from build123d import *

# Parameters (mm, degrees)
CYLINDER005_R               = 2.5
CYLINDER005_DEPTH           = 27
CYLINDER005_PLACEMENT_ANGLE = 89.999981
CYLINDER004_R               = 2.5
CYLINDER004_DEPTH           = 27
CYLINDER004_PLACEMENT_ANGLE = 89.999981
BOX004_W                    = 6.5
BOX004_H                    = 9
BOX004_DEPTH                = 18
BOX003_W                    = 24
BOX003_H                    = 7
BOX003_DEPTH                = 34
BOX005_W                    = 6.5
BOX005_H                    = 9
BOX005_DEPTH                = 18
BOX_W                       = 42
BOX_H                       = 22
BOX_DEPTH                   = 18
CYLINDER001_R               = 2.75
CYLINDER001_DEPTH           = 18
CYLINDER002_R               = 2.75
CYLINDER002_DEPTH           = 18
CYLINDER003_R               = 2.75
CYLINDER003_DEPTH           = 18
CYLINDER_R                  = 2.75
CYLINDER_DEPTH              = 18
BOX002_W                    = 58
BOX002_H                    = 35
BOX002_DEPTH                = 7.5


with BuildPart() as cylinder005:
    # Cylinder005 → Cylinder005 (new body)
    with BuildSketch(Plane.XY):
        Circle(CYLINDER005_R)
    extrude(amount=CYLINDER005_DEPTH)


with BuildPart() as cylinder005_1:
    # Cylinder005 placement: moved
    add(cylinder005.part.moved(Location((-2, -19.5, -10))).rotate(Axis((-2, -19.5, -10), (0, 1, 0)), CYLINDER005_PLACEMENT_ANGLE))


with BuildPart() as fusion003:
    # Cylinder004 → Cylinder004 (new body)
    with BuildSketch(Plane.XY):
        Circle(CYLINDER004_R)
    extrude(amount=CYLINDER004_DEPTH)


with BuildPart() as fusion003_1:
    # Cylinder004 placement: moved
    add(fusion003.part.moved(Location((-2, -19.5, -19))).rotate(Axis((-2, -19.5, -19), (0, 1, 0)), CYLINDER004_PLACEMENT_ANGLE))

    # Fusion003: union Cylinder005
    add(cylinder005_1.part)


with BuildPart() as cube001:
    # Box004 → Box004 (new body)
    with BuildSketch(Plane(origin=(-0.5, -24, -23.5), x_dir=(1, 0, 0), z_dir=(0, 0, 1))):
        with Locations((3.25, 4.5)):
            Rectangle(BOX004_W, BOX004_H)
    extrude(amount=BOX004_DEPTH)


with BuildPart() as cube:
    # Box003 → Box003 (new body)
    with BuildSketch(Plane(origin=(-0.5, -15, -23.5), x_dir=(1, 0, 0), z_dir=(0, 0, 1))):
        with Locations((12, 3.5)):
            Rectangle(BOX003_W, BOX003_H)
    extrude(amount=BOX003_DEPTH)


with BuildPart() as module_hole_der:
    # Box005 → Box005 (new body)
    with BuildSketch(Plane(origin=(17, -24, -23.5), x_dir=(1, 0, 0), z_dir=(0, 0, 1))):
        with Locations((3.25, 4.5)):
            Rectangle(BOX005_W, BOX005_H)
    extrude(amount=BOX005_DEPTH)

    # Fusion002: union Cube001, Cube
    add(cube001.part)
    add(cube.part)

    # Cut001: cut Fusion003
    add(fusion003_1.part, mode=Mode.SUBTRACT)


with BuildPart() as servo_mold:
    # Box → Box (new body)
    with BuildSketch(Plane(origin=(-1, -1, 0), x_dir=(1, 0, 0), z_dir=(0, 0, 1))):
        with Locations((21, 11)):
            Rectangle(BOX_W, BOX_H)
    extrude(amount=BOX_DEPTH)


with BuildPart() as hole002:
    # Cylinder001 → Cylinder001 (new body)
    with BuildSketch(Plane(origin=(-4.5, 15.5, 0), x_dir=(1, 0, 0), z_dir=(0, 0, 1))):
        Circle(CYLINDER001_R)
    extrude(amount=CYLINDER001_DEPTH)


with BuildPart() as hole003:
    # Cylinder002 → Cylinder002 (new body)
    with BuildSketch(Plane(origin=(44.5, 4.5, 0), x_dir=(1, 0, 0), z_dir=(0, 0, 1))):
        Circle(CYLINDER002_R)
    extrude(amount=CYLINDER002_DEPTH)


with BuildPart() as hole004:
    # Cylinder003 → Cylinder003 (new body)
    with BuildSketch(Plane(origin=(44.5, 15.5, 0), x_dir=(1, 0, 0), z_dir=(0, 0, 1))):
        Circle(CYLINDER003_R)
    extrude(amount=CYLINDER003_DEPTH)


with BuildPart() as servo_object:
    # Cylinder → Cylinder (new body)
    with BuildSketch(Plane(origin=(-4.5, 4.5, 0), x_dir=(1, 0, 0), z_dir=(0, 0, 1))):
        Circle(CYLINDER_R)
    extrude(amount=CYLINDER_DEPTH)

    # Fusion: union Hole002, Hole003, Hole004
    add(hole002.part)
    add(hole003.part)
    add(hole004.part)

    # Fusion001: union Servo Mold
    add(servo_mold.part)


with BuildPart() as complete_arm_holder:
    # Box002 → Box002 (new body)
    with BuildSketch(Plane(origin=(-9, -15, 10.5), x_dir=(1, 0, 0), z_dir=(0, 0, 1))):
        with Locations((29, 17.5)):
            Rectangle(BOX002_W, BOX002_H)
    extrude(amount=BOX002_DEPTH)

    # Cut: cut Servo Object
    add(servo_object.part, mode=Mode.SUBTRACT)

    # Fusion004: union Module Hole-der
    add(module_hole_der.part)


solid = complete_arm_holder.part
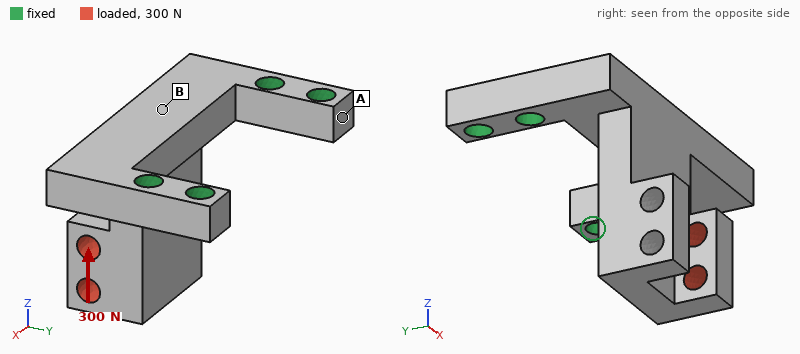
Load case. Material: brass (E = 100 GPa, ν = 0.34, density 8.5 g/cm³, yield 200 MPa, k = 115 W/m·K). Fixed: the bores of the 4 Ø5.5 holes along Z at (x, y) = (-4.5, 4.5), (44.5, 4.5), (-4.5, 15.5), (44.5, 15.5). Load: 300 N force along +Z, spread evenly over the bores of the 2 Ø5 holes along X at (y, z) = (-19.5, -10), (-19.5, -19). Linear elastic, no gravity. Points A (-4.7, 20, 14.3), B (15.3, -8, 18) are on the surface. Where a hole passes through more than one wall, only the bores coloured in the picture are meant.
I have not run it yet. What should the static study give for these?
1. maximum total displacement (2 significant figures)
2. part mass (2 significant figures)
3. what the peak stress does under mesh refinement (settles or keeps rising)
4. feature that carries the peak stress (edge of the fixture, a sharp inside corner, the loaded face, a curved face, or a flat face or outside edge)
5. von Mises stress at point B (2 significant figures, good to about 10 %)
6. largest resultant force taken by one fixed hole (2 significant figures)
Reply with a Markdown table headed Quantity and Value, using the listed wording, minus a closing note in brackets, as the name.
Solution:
| Quantity | Value |
|---|---|
| maximum total displacement | 83 µm |
| part mass | 130 g |
| what the peak stress does under mesh refinement | keeps rising |
| feature that carries the peak stress | edge of the fixture |
| von Mises stress at point B | 8.5 MPa |
| largest resultant force taken by one fixed hole | 160 N |
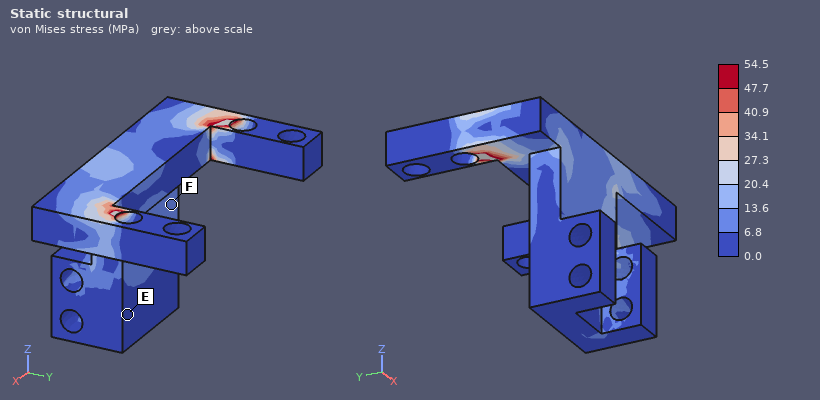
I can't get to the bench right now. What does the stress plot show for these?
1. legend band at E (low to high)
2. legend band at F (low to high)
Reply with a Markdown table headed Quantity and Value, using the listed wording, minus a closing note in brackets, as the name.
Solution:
| Quantity | Value |
|---|---|
| legend band at E | 0.0 to 6.8 MPa |
| legend band at F | 6.8 to 13.6 MPa |
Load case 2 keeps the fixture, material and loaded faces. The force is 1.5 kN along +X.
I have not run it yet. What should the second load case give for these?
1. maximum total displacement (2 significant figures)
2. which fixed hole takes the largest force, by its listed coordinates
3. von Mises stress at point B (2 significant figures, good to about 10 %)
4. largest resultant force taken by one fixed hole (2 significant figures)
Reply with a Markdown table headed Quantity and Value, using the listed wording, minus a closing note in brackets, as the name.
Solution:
| Quantity | Value |
|---|---|
| maximum total displacement | 0.17 mm |
| which fixed hole takes the largest force, by its listed coordinates | (44.5, 4.5) |
| von Mises stress at point B | 43 MPa |
| largest resultant force taken by one fixed hole | 1.4 kN |
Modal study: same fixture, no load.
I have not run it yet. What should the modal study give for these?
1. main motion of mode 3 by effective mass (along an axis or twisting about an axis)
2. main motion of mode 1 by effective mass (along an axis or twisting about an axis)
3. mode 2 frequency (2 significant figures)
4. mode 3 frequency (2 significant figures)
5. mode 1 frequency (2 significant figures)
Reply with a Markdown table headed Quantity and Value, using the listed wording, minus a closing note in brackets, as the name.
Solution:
| Quantity | Value |
|---|---|
| main motion of mode 3 by effective mass | along Z |
| main motion of mode 1 by effective mass | along Y |
| mode 2 frequency | 2800 Hz |
| mode 3 frequency | 4400 Hz |
| mode 1 frequency | 1200 Hz |
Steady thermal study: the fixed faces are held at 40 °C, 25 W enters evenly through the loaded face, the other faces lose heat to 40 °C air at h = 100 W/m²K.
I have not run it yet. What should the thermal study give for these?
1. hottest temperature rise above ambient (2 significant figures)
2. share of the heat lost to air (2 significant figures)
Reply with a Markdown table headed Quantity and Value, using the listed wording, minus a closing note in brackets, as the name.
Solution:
| Quantity | Value |
|---|---|
| hottest temperature rise above ambient | 56 K |
| share of the heat lost to air | 50 % |
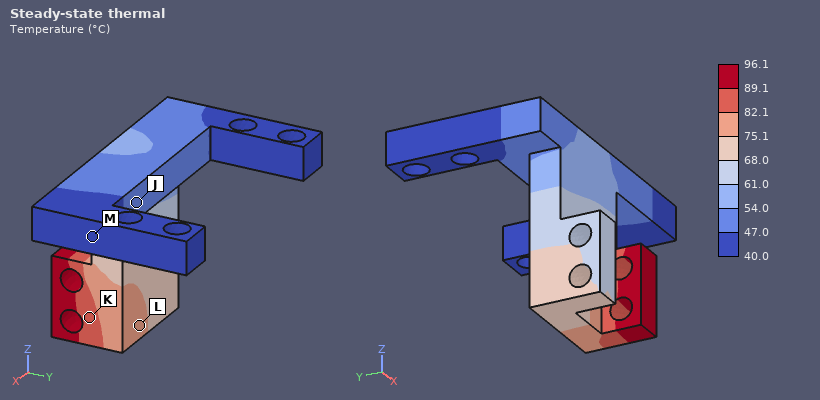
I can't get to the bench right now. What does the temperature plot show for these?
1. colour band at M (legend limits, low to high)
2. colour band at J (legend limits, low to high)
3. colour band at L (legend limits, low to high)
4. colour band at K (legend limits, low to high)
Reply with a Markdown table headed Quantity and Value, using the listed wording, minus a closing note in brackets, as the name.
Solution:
| Quantity | Value |
|---|---|
| colour band at M | 40.0 to 47.0 °C |
| colour band at J | 47.0 to 54.0 °C |
| colour band at L | 75.1 to 82.1 °C |
| colour band at K | 82.1 to 89.1 °C |
